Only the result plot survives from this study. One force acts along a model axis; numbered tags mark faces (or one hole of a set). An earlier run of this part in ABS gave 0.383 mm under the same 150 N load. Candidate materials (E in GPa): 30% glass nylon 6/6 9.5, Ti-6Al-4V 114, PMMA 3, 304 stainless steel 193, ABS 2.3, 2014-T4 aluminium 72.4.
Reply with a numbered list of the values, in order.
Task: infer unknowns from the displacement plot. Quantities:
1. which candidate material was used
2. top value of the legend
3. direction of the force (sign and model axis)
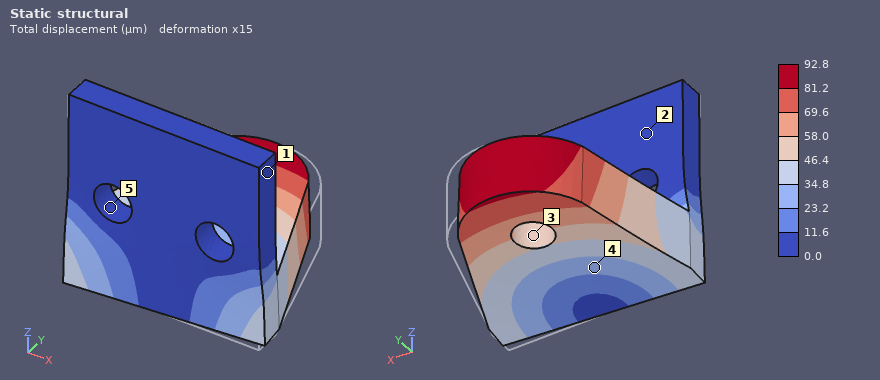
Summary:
1. 30% glass nylon 6/6
2. 92.8 µm
3. -X
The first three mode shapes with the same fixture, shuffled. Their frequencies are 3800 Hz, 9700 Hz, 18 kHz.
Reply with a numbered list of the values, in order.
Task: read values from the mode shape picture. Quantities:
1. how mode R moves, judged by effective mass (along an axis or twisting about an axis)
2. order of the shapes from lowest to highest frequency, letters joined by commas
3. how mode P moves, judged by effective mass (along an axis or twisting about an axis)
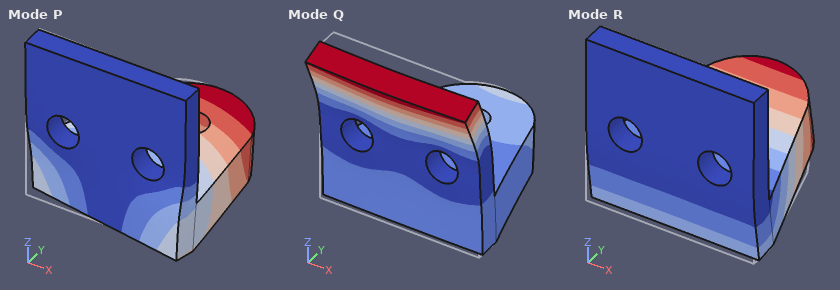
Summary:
1. along Z
2. R, P, Q
3. along X
